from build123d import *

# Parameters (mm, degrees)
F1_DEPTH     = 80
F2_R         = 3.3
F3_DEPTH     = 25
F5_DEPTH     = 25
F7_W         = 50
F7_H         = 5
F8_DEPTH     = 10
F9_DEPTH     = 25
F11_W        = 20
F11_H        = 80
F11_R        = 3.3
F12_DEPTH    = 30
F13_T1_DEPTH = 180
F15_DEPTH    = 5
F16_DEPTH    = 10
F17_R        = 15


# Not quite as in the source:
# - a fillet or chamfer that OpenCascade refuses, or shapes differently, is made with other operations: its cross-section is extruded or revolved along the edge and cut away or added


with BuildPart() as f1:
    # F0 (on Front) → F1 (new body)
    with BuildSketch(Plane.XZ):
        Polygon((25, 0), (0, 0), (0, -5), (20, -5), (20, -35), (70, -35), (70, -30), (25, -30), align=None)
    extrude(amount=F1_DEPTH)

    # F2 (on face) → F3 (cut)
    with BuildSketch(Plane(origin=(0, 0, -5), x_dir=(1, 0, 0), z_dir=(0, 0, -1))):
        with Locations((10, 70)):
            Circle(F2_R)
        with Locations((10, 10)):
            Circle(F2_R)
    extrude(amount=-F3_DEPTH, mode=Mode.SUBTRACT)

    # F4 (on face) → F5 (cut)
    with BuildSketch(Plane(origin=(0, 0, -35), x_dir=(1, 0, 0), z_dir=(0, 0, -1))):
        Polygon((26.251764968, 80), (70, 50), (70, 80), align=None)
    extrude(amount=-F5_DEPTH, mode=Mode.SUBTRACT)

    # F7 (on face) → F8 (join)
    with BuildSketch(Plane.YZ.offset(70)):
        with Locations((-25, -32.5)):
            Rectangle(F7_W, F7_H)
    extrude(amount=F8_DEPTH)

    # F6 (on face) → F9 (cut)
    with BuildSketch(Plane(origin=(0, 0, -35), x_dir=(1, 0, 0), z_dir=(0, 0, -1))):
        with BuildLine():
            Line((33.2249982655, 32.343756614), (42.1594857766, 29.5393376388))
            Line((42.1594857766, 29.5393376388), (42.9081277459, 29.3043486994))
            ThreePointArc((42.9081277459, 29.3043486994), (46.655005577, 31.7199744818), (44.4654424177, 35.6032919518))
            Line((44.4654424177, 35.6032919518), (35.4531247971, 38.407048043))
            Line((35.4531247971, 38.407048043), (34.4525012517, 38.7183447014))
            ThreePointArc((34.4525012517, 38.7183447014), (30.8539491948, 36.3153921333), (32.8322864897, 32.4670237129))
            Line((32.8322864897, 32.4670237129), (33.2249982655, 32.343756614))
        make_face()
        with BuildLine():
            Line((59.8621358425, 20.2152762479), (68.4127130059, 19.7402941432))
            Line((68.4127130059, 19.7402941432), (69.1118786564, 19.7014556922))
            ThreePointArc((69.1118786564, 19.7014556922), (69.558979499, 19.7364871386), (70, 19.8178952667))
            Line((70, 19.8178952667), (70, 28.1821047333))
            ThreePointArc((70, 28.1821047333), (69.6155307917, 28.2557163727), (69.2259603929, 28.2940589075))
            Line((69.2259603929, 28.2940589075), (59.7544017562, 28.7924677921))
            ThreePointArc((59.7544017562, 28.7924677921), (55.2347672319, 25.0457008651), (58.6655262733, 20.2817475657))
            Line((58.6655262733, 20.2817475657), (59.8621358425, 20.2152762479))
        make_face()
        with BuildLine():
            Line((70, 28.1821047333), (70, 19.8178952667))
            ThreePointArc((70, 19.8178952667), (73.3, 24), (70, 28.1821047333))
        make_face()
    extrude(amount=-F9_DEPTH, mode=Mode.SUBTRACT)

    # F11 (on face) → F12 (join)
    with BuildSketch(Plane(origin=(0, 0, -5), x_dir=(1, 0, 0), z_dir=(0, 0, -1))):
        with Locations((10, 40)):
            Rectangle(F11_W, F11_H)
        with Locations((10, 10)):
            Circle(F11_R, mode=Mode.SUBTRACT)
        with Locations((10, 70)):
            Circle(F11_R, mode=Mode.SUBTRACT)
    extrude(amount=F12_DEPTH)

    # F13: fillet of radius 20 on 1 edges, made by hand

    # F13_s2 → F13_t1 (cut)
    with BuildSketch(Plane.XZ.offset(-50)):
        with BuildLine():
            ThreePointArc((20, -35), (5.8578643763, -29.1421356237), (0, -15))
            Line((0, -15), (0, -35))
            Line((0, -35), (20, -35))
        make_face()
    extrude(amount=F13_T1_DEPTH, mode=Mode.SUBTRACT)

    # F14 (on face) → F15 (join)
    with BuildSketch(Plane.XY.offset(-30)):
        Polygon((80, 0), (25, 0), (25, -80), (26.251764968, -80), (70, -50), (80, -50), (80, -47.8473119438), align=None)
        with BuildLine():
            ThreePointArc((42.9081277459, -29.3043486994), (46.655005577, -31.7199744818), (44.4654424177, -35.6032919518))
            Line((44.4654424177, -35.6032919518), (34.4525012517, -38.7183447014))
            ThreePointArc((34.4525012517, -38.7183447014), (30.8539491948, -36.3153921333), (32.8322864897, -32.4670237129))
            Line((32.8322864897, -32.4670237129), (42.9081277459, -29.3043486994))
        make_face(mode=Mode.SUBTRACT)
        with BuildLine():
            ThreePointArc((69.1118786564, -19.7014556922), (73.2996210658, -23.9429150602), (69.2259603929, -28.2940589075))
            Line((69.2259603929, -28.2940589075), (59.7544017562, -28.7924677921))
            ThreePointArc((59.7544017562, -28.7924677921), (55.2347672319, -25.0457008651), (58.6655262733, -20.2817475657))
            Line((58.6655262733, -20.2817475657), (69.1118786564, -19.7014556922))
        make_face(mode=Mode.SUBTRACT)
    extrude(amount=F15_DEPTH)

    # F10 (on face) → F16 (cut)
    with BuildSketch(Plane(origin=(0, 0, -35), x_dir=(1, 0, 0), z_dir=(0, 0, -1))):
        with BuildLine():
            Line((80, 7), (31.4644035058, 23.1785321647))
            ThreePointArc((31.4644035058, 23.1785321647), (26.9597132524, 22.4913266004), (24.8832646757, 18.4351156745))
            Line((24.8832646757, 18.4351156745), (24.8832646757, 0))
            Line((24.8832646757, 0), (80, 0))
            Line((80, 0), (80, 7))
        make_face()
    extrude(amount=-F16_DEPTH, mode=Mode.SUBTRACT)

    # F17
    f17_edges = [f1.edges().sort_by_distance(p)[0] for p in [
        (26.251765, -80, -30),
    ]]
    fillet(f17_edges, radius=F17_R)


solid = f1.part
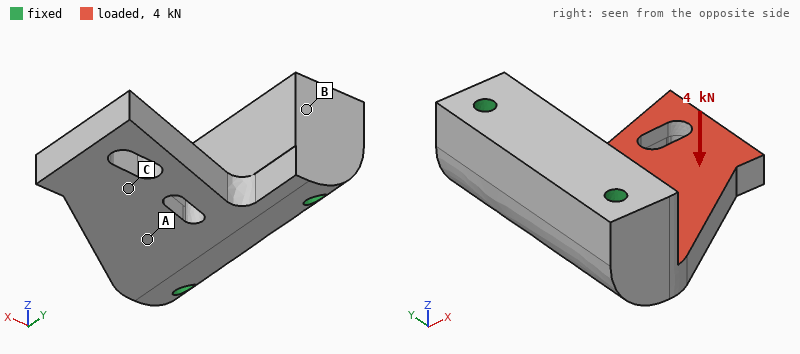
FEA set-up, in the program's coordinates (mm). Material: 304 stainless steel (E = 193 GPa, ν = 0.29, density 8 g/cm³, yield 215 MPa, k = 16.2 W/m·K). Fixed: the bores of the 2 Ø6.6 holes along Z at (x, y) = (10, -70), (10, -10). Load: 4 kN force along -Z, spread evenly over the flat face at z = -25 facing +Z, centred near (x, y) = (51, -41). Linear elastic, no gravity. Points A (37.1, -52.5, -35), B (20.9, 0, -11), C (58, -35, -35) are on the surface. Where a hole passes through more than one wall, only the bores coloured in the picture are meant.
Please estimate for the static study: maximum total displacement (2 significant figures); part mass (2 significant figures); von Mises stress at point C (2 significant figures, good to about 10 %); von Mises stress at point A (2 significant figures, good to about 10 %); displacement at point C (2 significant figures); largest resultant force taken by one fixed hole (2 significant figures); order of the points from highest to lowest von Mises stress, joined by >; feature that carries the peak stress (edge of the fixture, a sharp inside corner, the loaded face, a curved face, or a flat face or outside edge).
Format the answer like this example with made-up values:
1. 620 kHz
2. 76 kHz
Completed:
1. 0.20 mm
2. 670 g
3. 32 MPa
4. 79 MPa
5. 0.095 mm
6. 2.1 kN
7. A > C > B
8. a curved face
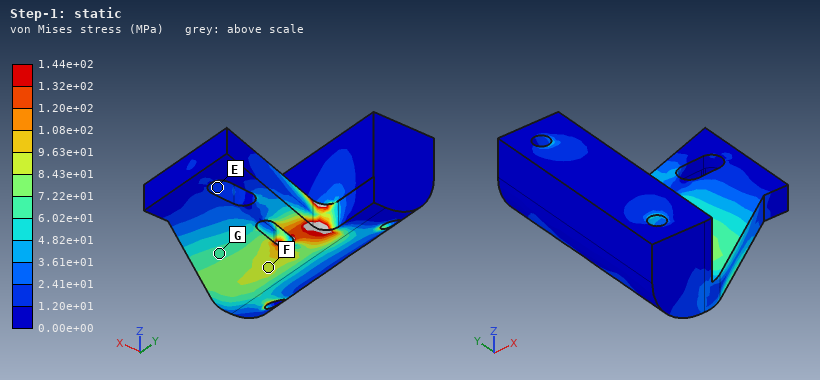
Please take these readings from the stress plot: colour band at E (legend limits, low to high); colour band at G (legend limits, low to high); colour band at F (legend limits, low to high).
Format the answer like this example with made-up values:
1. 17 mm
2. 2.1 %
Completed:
1. 1.20e+01 to 2.41e+01 MPa
2. 6.02e+01 to 7.22e+01 MPa
3. 8.43e+01 to 9.63e+01 MPa
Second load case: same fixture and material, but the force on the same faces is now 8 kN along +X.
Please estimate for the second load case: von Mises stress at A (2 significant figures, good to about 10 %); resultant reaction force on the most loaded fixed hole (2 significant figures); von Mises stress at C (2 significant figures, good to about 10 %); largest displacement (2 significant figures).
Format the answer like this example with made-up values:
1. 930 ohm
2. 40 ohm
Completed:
1. 30 MPa
2. 4.5 kN
3. 16 MPa
4. 67 µm
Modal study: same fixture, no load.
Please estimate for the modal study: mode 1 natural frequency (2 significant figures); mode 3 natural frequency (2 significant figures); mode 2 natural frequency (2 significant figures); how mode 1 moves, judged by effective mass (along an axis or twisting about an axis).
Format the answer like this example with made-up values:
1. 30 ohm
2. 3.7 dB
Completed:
1. 2200 Hz
2. 6600 Hz
3. 6000 Hz
4. along Z
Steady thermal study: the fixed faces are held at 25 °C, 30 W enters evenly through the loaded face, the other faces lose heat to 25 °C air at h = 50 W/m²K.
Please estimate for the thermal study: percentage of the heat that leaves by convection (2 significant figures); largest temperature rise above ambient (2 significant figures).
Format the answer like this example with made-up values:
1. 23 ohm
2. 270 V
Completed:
1. 51 %
2. 75 K
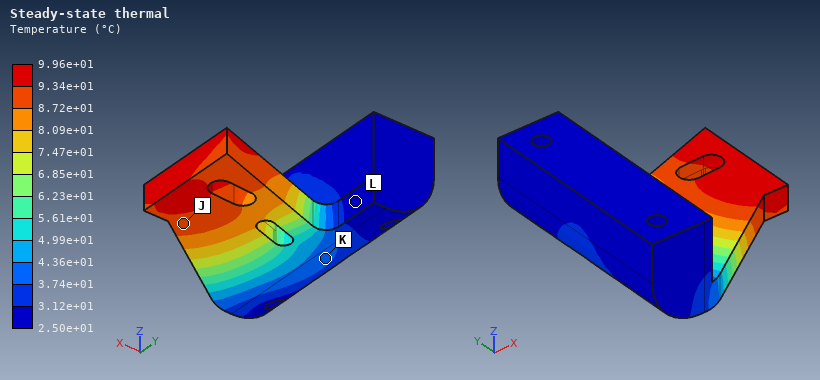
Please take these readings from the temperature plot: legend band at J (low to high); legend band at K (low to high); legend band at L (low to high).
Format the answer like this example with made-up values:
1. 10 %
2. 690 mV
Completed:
1. 8.72e+01 to 9.34e+01 °C
2. 3.74e+01 to 4.36e+01 °C
3. 2.50e+01 to 3.12e+01 °C
